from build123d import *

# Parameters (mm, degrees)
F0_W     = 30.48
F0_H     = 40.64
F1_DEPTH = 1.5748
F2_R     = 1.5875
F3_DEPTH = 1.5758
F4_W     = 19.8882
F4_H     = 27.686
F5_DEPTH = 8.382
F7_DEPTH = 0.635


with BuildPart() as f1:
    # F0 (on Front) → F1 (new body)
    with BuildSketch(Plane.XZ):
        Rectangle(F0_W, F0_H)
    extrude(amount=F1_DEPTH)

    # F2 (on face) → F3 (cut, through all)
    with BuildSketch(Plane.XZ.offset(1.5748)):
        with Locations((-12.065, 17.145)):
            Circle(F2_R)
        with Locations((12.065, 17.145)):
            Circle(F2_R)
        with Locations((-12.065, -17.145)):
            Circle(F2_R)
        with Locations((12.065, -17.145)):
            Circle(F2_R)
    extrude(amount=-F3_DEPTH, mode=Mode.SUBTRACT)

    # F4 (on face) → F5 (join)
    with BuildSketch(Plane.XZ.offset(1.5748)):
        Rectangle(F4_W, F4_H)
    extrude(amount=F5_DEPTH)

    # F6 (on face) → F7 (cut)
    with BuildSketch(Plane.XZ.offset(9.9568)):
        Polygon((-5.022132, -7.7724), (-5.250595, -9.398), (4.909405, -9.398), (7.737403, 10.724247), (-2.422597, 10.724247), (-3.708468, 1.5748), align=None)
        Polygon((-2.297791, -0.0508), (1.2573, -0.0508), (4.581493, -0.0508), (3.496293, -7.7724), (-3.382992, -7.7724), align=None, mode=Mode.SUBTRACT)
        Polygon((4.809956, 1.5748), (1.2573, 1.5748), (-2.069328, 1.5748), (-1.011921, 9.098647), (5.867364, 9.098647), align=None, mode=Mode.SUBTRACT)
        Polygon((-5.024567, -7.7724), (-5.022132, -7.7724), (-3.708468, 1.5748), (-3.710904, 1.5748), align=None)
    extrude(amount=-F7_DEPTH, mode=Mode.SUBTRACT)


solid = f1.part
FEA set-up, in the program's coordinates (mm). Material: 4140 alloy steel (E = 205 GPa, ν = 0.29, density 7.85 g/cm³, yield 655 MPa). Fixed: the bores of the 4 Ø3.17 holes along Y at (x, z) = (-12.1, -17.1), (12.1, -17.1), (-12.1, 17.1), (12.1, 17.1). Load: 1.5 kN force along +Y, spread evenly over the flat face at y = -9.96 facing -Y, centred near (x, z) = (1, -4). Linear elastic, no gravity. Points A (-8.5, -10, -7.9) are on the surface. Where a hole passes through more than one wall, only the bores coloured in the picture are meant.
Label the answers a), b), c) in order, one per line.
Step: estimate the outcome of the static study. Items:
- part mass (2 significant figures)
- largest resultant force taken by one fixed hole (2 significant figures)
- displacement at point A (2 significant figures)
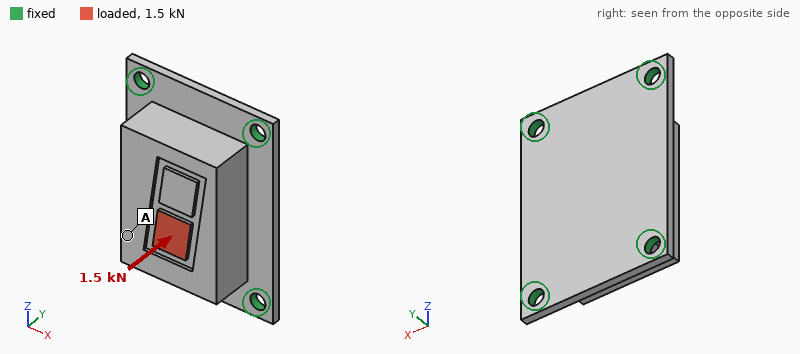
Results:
a) 51 g
b) 570 N
c) 9.8 µm
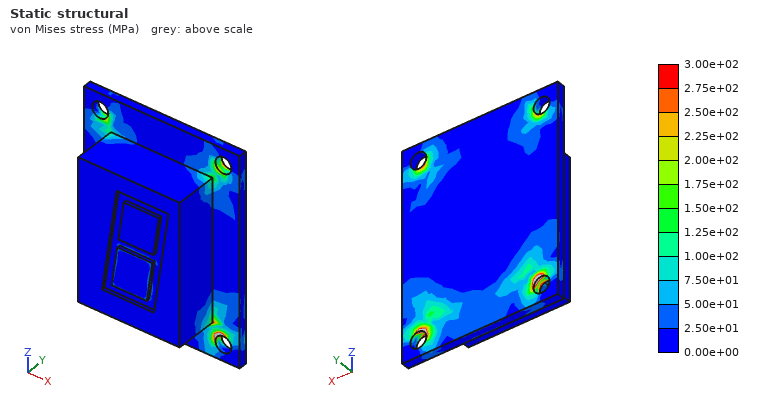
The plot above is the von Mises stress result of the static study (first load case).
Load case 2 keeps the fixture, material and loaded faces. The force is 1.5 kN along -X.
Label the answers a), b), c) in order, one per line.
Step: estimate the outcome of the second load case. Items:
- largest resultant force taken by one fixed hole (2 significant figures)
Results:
a) 600 N
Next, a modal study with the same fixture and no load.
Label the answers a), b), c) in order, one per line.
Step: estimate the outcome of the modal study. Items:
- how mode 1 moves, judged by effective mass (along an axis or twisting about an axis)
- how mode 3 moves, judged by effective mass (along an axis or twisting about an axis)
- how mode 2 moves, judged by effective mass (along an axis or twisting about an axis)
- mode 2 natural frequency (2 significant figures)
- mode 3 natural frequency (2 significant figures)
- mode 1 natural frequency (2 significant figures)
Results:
a) along Y
b) along Z
c) along X
d) 12 kHz
e) 15 kHz
f) 9500 Hz
